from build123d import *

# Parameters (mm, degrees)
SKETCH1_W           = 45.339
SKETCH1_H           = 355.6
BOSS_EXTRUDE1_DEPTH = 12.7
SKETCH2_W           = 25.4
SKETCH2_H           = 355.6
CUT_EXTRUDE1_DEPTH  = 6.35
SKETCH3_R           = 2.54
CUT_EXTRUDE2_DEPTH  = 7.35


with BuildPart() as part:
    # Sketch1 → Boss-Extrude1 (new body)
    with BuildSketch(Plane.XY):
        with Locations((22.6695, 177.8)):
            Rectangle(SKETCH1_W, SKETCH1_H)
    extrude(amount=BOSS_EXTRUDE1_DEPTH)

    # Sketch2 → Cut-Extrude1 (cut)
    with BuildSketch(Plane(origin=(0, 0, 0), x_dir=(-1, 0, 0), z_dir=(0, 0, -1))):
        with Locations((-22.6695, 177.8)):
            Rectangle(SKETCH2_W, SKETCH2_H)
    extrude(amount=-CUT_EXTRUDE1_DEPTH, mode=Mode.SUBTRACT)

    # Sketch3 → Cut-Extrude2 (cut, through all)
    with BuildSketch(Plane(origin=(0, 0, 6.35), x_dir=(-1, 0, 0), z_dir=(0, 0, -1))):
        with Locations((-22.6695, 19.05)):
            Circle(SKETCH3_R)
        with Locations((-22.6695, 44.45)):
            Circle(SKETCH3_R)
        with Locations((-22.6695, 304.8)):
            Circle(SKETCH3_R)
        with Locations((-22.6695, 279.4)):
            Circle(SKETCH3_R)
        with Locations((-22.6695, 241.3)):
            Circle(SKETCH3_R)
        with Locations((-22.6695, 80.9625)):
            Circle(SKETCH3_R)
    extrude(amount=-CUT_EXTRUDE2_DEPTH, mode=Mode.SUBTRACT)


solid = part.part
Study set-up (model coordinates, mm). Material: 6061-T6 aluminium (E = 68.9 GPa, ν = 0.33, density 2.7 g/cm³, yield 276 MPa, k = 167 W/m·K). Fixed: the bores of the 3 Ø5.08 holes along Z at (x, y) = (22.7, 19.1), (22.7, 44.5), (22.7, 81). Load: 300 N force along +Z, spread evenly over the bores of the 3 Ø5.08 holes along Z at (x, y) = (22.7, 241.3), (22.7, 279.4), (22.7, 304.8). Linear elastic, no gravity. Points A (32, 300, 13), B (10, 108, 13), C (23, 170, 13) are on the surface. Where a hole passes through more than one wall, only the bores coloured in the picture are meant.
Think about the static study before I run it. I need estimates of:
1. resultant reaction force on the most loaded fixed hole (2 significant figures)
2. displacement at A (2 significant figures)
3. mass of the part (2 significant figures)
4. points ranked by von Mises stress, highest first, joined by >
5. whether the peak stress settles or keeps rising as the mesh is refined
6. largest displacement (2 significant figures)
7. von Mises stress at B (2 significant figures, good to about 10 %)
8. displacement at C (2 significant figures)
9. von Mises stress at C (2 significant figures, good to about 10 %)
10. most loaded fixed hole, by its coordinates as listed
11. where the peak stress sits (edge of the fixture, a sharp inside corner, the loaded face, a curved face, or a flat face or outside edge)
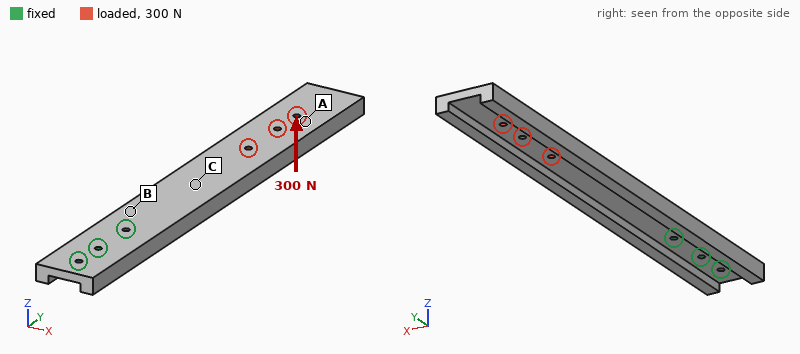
2.1 kN
3.0 mm
400 g
B > C > A
keeps rising
4.0 mm
51 MPa
0.75 mm
32 MPa
(22.7, 81)
edge of the fixture
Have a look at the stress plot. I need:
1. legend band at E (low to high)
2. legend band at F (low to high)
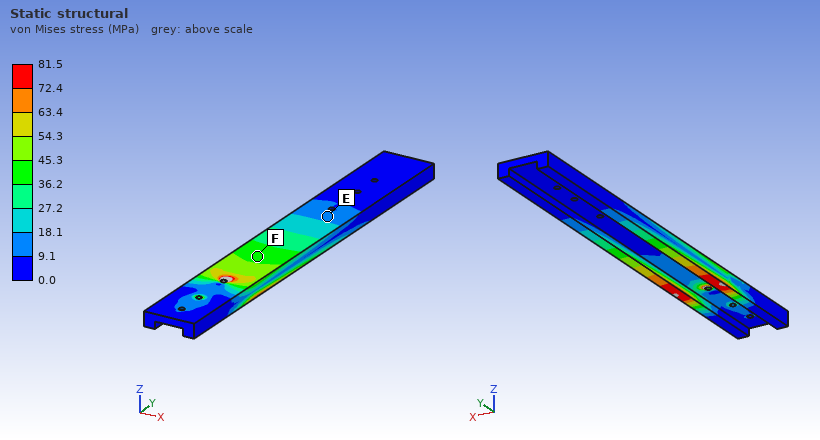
9.1 to 18.1 MPa
36.2 to 45.3 MPa
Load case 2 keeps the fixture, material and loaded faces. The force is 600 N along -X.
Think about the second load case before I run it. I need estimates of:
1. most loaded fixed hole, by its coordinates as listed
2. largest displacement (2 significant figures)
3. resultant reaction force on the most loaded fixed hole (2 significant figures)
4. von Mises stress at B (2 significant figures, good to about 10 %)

(22.7, 81)
0.59 mm
2.8 kN
15 MPa
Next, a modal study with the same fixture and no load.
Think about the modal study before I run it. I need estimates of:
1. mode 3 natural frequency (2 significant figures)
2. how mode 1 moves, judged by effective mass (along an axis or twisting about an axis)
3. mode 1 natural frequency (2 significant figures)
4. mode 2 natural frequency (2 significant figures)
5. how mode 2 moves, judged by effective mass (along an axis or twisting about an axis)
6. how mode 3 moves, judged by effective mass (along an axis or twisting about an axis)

750 Hz
along Z
120 Hz
440 Hz
along X
along Z
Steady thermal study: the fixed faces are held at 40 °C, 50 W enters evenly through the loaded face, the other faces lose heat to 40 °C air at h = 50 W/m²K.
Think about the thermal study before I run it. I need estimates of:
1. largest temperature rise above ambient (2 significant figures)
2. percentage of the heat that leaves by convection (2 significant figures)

43 K
83 %
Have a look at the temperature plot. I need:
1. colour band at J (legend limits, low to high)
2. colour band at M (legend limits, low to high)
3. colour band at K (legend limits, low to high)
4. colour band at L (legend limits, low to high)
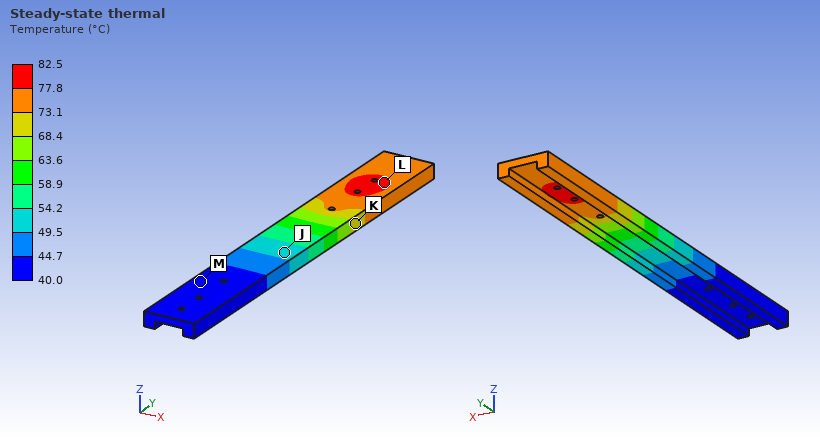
49.5 to 54.2 °C
40.0 to 44.7 °C
68.4 to 73.1 °C
77.8 to 82.5 °C
